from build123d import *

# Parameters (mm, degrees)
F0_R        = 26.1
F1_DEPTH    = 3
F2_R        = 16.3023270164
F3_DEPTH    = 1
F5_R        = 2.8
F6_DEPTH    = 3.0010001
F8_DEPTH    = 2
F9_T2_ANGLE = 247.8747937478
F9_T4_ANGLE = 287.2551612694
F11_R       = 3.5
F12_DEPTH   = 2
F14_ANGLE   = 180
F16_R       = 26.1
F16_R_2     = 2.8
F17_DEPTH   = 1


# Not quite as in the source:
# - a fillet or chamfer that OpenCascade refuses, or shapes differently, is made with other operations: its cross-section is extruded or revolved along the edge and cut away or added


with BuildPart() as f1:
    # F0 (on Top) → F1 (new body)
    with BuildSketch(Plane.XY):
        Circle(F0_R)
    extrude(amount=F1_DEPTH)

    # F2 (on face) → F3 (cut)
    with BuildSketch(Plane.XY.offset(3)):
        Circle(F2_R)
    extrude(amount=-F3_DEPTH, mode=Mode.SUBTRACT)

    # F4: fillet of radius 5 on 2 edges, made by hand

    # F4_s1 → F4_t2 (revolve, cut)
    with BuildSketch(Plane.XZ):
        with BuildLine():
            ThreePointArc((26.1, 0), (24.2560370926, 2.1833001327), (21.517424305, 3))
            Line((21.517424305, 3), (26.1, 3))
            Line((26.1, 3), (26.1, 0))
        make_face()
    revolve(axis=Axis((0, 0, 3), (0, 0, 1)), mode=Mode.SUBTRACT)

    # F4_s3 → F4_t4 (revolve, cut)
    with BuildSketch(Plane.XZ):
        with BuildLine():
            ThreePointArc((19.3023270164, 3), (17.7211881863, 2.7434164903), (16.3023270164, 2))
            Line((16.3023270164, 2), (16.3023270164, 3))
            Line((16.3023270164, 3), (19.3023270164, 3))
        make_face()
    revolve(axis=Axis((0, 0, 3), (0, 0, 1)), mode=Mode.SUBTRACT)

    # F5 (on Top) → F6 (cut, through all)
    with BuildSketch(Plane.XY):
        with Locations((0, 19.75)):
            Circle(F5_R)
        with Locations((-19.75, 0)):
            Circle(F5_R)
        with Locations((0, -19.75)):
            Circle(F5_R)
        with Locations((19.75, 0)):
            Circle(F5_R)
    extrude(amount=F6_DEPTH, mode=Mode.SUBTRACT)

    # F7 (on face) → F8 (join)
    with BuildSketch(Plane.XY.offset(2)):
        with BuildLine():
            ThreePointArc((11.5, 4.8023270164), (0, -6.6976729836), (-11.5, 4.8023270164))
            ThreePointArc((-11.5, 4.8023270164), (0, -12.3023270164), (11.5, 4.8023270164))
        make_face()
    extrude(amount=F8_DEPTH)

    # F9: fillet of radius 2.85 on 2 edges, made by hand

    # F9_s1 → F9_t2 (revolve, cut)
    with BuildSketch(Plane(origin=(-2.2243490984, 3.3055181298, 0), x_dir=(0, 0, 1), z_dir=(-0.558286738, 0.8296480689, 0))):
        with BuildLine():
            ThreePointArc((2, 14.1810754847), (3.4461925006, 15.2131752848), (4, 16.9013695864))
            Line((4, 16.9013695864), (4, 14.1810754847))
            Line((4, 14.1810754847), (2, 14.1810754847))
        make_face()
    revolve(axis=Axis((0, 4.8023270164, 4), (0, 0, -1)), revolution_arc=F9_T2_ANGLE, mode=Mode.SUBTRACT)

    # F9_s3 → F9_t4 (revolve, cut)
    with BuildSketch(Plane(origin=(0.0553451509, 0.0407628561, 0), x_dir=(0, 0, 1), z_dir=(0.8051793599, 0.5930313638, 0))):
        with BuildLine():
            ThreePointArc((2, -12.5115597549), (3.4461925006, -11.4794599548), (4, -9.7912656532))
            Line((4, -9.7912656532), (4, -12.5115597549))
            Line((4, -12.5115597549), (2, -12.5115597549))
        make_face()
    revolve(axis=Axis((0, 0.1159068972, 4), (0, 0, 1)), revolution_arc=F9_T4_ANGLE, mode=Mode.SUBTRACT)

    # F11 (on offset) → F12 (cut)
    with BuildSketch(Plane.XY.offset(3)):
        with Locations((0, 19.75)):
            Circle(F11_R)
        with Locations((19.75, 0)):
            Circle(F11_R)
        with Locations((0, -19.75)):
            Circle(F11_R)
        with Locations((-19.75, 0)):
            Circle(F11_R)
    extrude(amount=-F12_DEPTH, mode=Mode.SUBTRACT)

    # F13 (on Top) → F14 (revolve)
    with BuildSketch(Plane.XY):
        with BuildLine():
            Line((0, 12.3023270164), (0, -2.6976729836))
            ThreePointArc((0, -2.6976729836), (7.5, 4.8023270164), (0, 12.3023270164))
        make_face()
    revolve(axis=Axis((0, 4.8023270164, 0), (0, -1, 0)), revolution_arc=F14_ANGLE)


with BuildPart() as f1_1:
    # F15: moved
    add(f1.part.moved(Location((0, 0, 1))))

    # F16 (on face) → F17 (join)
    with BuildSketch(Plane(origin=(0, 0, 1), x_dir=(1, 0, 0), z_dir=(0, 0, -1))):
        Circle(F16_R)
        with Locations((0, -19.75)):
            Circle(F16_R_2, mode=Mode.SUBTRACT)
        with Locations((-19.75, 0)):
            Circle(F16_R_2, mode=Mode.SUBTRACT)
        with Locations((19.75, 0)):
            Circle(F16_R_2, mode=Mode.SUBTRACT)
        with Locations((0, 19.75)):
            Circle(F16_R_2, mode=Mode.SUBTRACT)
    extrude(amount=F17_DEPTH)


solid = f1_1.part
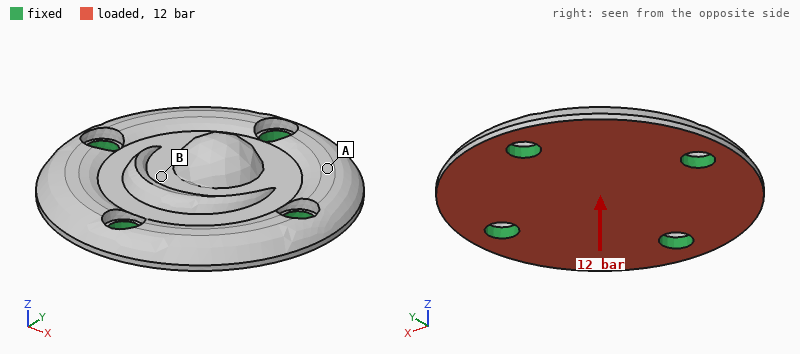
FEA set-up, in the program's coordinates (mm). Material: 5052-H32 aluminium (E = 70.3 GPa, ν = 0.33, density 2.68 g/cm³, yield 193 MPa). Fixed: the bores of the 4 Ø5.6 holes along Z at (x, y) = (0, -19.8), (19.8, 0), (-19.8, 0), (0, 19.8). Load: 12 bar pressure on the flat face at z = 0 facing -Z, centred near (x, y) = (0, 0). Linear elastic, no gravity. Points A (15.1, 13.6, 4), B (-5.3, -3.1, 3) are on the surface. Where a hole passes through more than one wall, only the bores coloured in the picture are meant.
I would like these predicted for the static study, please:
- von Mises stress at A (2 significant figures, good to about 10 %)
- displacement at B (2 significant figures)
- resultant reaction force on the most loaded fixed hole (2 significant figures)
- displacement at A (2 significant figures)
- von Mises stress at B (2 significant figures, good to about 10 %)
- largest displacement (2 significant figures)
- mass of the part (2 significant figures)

29 MPa
12 µm
660 N
14 µm
14 MPa
21 µm
19 g
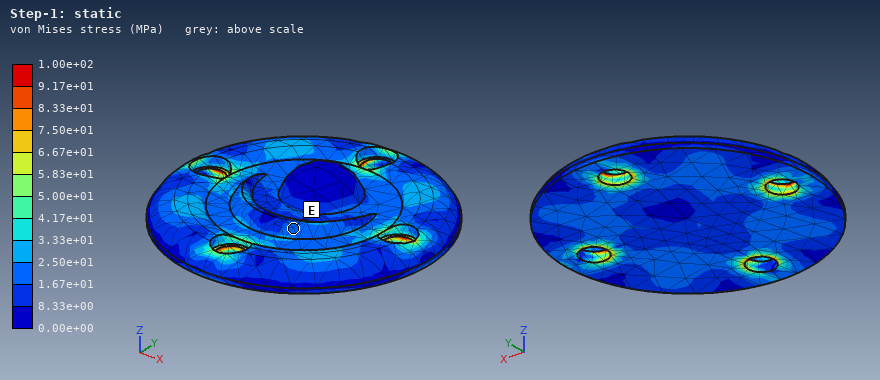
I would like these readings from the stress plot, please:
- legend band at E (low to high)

1.67e+01 to 2.50e+01 MPa
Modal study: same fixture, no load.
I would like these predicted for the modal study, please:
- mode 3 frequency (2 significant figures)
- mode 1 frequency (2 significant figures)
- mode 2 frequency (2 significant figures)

16 kHz
16 kHz
16 kHz
